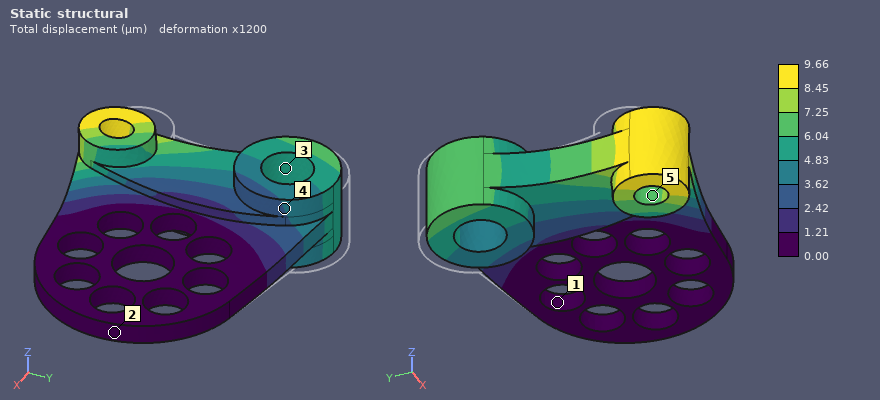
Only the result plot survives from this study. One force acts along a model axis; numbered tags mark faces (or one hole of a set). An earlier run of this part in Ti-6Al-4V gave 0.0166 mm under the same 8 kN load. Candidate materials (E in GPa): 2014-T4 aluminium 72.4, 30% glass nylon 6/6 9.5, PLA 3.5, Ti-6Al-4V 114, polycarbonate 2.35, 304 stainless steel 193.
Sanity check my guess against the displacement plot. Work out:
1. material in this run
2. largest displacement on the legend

304 stainless steel
9.66 µm
